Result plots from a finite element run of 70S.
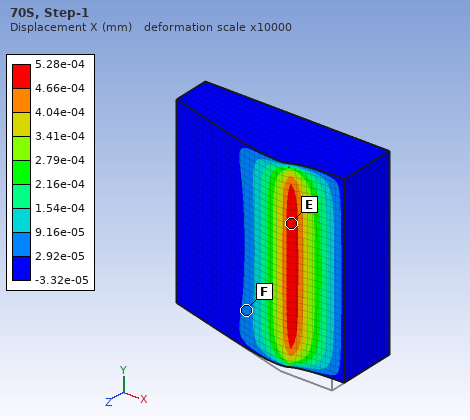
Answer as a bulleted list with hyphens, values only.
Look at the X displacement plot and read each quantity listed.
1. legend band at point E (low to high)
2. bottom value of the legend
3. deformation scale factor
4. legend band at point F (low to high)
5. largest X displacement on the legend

- 4.66e-04 to 5.28e-04 mm
- -3.32e-05 mm
- 10000
- 2.92e-05 to 9.16e-05 mm
- 5.28e-04 mm
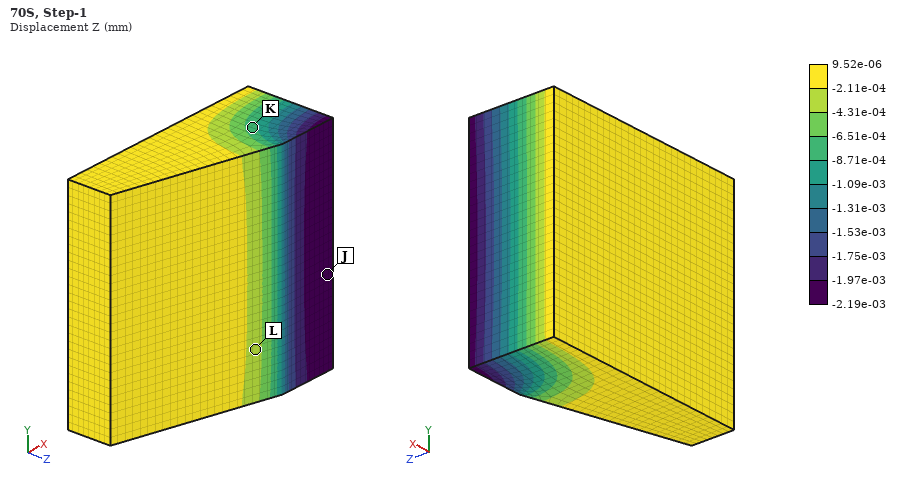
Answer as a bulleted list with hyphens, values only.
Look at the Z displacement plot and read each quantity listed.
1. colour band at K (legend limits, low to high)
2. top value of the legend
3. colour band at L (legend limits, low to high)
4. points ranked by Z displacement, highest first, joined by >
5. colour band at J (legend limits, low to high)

- -8.71e-04 to -6.51e-04 mm
- 9.52e-06 mm
- -4.31e-04 to -2.11e-04 mm
- L > K > J
- -2.19e-03 to -1.97e-03 mm
